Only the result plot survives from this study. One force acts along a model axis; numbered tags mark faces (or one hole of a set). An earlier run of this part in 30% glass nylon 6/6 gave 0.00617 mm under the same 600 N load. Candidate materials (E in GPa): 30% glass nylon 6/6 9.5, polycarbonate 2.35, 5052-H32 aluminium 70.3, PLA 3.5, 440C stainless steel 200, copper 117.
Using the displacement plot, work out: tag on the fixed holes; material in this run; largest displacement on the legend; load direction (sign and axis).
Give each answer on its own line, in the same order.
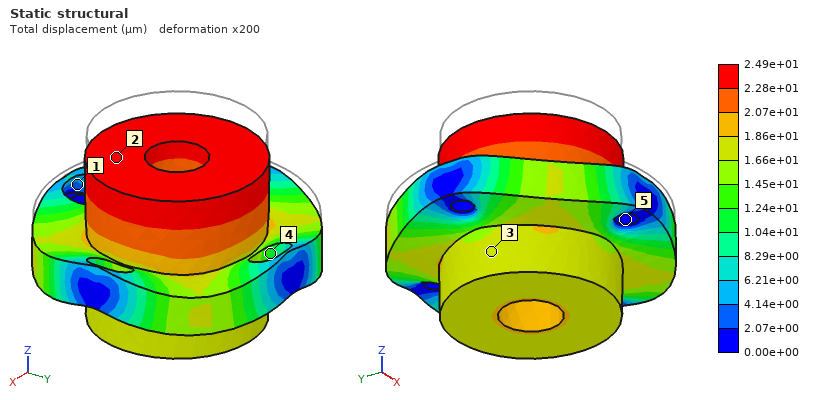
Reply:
5
polycarbonate
2.49e+01 µm
-Z
